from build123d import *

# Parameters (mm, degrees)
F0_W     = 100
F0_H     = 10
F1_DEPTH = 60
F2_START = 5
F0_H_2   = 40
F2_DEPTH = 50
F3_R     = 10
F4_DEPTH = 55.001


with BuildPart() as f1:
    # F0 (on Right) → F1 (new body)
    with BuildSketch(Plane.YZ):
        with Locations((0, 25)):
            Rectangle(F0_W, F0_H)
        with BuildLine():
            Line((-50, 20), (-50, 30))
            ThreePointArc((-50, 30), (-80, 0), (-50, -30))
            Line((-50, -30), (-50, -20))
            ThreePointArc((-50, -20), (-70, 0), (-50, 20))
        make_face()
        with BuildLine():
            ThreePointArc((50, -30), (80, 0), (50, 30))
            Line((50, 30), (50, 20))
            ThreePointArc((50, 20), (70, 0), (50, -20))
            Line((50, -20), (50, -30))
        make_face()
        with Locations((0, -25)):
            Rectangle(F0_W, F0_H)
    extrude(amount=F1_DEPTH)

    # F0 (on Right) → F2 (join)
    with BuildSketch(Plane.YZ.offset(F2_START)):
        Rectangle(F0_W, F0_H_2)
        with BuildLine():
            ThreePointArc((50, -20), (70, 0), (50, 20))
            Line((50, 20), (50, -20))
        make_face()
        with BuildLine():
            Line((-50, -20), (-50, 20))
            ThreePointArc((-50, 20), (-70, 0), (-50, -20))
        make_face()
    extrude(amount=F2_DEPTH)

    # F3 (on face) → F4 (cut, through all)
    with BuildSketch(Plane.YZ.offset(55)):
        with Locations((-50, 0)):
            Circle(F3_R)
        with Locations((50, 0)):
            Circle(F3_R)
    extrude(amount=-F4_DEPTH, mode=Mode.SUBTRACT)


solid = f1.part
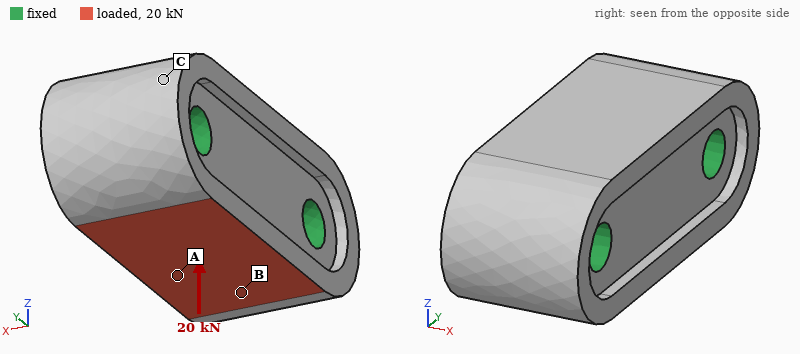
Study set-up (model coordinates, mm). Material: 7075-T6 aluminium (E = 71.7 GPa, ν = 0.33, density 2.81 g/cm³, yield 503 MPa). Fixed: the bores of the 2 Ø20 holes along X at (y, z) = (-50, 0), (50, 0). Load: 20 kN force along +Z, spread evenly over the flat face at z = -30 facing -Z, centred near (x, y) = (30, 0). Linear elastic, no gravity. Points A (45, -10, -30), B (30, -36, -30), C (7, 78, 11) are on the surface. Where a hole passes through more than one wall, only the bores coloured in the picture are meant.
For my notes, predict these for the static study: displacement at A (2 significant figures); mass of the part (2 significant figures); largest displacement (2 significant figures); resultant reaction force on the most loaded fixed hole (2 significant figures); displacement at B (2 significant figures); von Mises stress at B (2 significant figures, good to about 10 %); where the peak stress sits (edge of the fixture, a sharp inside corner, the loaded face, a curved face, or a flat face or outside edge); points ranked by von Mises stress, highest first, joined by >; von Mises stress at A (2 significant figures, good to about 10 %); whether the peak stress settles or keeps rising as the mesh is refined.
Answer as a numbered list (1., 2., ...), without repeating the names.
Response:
1. 4.9 µm
2. 1.3 kg
3. 6.7 µm
4. 10 kN
5. 2.7 µm
6. 4.0 MPa
7. edge of the fixture
8. A > B > C
9. 6.4 MPa
10. keeps rising
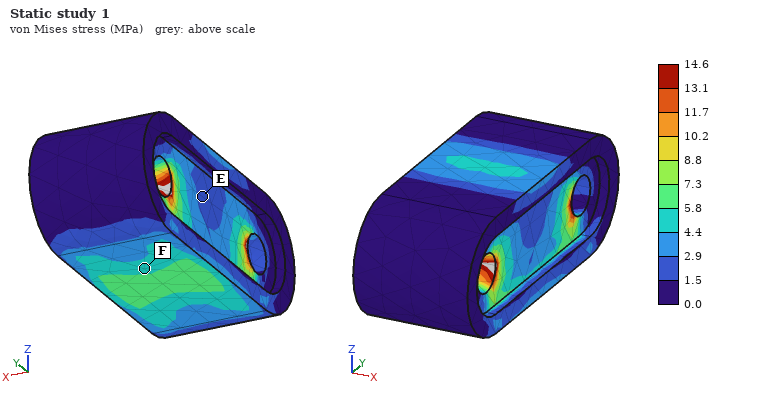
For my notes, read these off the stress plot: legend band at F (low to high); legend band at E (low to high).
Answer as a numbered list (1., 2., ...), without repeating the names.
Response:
1. 4.4 to 5.8 MPa
2. 1.5 to 2.9 MPa
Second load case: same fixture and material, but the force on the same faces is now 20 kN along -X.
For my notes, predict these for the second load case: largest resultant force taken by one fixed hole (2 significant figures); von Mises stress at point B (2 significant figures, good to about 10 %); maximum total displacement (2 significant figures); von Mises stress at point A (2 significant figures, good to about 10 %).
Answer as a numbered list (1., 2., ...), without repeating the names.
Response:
1. 10 kN
2. 13 MPa
3. 17 µm
4. 8.9 MPa
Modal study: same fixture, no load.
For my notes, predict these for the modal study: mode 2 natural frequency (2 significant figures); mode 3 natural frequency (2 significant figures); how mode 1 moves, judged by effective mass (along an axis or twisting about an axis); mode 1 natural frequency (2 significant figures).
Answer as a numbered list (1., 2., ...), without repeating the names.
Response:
1. 13 kHz
2. 13 kHz
3. along Z
4. 13 kHz
